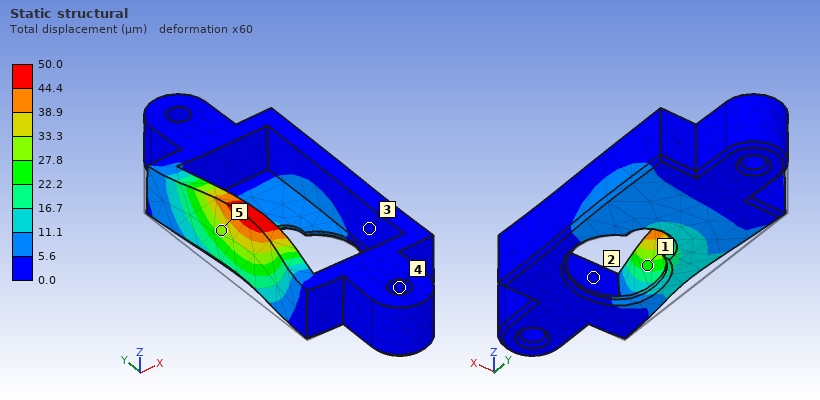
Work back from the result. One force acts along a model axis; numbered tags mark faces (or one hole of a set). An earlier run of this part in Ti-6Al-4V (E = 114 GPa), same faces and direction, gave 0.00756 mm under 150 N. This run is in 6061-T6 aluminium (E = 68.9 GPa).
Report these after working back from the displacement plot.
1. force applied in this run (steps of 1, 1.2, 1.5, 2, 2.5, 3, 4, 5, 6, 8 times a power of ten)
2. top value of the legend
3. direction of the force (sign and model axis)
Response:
600 N
50.0 µm
+X
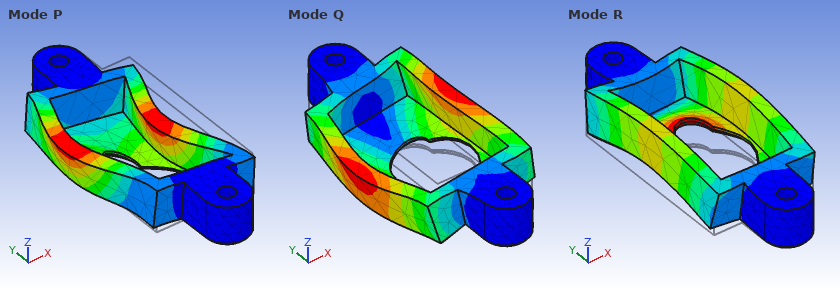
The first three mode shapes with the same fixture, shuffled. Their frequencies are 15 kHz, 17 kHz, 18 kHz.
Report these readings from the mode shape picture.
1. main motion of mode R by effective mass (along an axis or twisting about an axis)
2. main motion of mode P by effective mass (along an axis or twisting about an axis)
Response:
along Z
along X
